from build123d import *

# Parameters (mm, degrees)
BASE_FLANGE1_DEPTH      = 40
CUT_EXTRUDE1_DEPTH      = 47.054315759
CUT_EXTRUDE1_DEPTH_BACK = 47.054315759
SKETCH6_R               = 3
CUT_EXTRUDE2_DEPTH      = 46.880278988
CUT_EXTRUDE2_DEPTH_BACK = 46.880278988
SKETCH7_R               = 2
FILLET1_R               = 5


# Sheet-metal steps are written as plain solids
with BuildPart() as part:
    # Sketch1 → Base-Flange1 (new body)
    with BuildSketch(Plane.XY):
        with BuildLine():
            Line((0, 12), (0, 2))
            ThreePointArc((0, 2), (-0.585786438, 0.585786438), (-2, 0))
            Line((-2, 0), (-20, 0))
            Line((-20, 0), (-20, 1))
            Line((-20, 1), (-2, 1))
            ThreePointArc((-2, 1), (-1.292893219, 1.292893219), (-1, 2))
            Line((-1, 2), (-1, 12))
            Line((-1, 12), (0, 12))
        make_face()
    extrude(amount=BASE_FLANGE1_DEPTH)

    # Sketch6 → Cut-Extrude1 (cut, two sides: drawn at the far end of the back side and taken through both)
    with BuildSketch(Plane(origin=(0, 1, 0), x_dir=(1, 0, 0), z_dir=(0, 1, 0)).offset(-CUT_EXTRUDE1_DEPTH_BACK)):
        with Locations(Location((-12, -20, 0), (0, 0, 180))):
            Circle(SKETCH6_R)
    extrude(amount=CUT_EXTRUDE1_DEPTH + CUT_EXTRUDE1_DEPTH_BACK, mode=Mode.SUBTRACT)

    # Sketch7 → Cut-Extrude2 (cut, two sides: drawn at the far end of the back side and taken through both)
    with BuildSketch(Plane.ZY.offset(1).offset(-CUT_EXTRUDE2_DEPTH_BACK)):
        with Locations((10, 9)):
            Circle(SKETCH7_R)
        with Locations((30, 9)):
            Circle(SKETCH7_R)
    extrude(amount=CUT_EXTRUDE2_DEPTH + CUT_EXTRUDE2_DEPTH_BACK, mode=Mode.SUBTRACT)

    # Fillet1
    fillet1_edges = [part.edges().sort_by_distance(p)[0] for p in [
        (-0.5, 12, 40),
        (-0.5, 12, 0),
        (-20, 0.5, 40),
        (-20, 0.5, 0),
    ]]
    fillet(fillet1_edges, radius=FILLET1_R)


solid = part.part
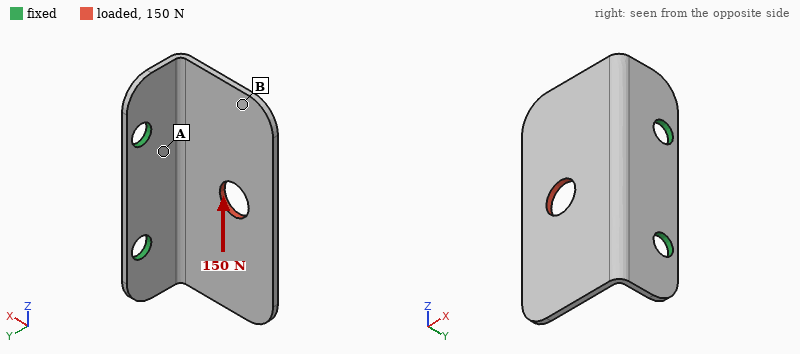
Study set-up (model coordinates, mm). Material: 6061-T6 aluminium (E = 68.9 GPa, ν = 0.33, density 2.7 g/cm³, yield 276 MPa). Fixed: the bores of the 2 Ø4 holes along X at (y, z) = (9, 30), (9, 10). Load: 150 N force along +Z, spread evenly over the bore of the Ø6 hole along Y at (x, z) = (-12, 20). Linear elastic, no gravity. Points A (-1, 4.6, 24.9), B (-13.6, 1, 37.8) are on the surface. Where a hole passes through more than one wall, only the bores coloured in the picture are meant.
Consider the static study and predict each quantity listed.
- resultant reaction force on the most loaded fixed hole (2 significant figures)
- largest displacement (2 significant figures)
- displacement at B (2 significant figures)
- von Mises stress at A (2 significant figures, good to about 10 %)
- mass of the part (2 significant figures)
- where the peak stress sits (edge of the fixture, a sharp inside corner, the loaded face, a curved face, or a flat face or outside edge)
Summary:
120 N
0.23 mm
0.19 mm
62 MPa
3.1 g
a flat face or outside edge
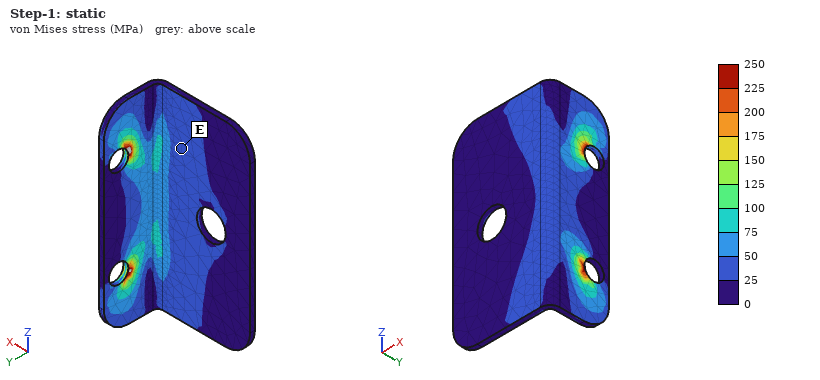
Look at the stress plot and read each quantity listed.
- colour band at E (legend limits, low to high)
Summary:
25 to 50 MPa
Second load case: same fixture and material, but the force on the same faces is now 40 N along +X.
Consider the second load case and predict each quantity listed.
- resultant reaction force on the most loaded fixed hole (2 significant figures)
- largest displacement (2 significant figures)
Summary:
20 N
0.11 mm
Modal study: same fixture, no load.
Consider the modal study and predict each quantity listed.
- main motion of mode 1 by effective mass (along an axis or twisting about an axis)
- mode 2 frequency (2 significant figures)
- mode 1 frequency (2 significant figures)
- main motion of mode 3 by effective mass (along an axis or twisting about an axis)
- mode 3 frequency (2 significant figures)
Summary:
along Y
2400 Hz
1400 Hz
along Z
4300 Hz
